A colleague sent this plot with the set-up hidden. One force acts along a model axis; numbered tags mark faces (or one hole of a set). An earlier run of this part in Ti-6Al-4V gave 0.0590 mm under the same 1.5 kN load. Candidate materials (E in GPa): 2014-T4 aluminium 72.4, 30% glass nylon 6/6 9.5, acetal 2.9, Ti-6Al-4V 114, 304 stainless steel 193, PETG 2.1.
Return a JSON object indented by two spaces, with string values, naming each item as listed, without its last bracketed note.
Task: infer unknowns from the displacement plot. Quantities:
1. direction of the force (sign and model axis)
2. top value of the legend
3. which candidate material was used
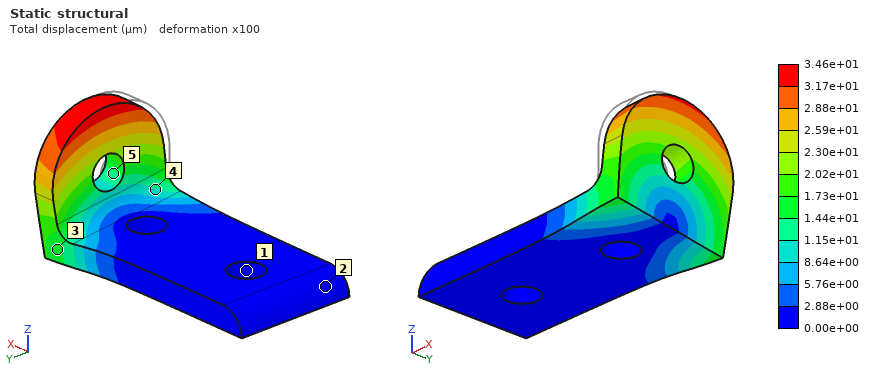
{
  "direction of the force": "+Y",
  "top value of the legend": "3.46e+01 µm",
  "which candidate material was used": "304 stainless steel"
}
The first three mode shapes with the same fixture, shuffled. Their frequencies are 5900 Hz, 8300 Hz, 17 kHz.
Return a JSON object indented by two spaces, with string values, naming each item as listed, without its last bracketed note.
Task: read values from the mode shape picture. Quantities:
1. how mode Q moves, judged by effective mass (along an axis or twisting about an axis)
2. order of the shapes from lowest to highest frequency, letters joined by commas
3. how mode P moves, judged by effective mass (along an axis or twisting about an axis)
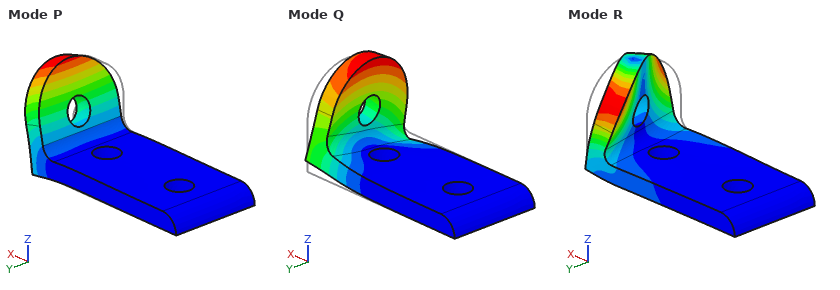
{
  "how mode Q moves, judged by effective mass": "along Y",
  "order of the shapes from lowest to highest frequency, letters joined by commas": "P, Q, R",
  "how mode P moves, judged by effective mass": "along X"
}
